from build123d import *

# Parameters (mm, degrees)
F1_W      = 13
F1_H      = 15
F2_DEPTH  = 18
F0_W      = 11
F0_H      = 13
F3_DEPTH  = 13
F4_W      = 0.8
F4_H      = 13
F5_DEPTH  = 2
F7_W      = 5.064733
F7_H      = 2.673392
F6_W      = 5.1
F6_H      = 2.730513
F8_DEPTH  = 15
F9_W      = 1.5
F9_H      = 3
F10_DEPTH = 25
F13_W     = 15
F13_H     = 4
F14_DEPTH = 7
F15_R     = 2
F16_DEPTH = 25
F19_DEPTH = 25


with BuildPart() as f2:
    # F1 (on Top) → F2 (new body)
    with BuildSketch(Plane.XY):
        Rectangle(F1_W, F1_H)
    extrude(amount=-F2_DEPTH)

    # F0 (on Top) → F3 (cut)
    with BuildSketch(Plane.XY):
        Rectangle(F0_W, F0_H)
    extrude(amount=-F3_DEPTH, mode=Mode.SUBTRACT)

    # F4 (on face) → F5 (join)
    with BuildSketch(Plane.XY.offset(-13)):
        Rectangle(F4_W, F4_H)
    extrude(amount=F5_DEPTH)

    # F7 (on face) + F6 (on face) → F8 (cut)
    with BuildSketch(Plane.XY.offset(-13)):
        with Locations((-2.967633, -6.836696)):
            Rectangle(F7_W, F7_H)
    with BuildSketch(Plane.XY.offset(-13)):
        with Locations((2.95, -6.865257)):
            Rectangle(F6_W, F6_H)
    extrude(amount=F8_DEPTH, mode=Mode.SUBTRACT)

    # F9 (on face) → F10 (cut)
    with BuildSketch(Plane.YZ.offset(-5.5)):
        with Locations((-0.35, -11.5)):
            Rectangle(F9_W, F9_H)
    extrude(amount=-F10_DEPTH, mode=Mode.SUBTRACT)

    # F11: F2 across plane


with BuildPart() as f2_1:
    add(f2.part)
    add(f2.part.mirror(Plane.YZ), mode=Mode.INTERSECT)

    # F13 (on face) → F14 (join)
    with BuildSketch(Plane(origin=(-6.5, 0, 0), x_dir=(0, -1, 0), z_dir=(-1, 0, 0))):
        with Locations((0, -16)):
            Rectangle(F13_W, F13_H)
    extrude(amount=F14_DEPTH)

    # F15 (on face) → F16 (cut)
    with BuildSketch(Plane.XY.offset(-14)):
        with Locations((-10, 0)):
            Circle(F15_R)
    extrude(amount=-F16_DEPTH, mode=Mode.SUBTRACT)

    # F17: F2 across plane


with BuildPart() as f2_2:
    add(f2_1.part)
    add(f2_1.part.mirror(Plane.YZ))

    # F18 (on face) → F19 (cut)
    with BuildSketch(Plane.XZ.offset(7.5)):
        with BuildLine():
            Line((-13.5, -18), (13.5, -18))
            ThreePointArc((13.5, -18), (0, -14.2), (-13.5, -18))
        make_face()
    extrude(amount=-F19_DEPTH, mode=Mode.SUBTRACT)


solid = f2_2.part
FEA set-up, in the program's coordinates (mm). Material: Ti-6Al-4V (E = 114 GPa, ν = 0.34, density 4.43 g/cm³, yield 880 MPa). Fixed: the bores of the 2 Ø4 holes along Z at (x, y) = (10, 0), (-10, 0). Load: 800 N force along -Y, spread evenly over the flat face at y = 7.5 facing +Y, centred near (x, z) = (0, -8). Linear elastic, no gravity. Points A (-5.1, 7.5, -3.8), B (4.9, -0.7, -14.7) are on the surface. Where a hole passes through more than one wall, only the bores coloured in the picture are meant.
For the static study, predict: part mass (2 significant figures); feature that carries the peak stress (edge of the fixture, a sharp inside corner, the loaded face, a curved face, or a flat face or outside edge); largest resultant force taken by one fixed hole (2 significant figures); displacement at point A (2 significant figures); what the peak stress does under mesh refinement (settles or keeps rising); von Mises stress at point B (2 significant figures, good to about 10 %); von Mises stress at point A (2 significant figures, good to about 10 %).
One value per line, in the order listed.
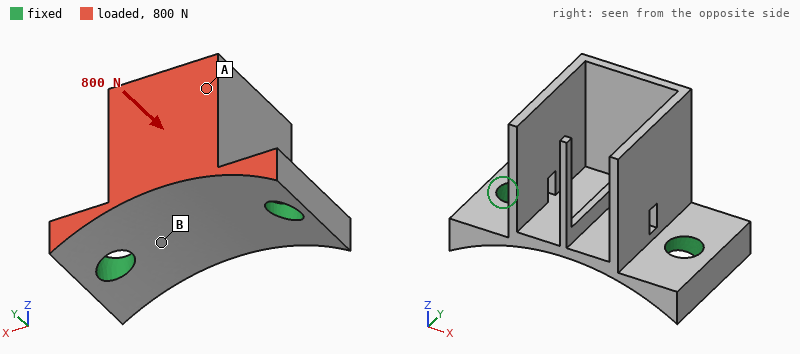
5.6 g
edge of the fixture
400 N
0.068 mm
keeps rising
27 MPa
75 MPa
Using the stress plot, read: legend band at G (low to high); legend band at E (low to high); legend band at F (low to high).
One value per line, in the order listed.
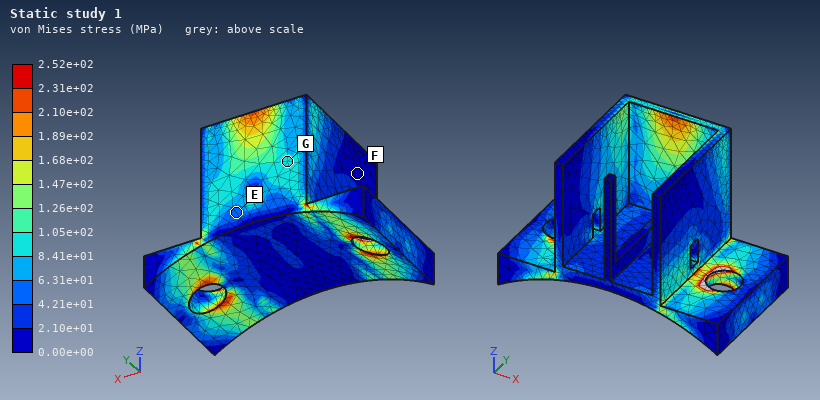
8.41e+01 to 1.05e+02 MPa
4.21e+01 to 6.31e+01 MPa
0.00e+00 to 2.10e+01 MPa
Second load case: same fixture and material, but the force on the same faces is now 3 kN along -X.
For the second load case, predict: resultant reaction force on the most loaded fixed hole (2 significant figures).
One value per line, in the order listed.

2.2 kN
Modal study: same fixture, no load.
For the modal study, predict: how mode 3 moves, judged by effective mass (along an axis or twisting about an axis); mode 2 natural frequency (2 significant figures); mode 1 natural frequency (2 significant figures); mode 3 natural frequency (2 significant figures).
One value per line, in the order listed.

along X
6000 Hz
4300 Hz
7000 Hz
